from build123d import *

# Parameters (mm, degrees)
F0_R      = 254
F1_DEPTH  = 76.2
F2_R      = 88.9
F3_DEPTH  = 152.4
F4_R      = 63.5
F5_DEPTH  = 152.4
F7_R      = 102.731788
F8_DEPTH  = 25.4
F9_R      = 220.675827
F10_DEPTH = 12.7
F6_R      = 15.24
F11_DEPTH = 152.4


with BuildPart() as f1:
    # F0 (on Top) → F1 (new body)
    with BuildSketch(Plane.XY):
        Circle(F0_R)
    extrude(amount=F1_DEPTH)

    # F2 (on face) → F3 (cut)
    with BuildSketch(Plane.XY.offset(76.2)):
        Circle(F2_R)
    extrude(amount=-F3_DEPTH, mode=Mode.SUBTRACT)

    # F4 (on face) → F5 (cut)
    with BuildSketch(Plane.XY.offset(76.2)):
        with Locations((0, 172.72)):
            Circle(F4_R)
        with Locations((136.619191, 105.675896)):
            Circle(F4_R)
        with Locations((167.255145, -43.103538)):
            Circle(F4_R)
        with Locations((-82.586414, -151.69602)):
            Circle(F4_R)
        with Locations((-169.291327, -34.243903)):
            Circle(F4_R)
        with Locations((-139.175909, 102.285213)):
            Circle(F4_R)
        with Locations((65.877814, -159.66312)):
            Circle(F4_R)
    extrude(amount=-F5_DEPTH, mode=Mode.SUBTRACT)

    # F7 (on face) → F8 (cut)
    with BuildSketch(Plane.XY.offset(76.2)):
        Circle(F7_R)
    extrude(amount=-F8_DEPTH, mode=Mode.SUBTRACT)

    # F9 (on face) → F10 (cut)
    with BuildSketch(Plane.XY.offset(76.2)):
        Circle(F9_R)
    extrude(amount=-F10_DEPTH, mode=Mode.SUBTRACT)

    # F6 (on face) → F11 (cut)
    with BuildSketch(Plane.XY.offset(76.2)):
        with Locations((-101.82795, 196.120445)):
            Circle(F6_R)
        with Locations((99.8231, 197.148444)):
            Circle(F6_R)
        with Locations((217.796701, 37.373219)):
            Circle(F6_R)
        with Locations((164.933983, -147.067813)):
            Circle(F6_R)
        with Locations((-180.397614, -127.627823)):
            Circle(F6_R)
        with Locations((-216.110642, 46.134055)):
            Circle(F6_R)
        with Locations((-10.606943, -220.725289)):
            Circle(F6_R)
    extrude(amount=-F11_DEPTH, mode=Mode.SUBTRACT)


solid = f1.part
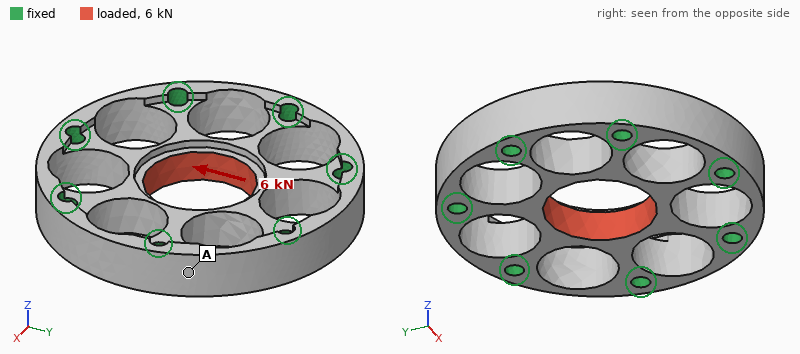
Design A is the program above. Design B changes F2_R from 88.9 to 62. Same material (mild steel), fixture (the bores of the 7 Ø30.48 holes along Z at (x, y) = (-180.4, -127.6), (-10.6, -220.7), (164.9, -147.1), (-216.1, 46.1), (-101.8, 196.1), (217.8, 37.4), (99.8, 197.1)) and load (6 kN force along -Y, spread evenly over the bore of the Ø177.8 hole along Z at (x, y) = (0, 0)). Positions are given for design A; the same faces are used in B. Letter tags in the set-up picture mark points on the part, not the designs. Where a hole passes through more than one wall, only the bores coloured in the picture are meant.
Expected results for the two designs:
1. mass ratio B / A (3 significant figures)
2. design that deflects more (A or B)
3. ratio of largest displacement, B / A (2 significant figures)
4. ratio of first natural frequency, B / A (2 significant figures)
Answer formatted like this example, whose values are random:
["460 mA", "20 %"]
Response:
["1.11", "A", "0.85", "0.81"]
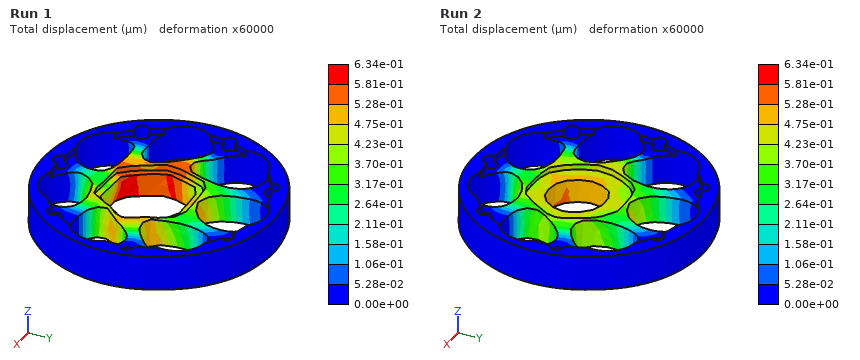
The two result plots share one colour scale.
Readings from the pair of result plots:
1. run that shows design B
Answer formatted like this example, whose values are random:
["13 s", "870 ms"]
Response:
["Run 2"]
